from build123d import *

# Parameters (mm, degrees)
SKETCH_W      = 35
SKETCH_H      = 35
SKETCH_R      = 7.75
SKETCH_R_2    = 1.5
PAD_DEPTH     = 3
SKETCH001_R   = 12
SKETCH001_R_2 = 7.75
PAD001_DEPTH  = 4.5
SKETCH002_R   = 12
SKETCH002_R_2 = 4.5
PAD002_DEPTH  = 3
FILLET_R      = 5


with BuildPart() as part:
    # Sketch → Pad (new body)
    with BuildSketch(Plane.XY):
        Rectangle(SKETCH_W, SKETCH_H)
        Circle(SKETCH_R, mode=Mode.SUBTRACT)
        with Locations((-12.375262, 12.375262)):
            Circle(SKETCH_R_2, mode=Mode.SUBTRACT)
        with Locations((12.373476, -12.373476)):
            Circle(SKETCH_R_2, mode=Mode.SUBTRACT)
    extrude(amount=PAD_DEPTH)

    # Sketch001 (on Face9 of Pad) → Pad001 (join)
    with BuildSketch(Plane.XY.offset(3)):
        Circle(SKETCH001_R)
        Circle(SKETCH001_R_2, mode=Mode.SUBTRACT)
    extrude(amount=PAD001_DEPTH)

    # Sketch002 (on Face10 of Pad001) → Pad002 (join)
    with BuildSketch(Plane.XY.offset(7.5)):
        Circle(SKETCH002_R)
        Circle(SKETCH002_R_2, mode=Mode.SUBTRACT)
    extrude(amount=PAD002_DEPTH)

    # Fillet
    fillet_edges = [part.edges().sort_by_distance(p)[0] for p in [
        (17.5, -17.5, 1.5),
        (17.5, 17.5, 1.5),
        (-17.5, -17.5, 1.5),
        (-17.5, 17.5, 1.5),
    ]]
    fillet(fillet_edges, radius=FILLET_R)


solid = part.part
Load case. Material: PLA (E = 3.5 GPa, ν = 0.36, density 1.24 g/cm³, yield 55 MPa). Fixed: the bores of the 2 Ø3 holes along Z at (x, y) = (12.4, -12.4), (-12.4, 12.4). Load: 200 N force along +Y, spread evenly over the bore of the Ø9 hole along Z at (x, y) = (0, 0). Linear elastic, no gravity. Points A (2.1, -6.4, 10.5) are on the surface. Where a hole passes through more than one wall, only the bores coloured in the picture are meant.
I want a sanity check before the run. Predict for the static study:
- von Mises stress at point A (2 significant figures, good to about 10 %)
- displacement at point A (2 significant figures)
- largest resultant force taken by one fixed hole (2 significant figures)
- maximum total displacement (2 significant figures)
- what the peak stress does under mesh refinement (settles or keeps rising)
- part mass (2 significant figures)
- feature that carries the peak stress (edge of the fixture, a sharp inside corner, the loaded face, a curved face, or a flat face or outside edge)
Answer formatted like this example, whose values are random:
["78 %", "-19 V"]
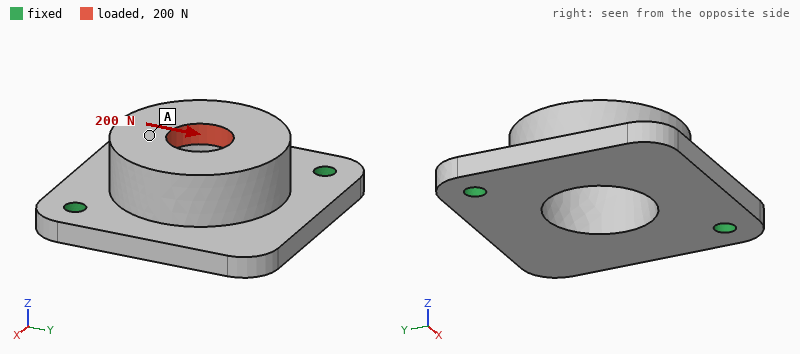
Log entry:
["3.8 MPa", "0.18 mm", "110 N", "0.40 mm", "keeps rising", "6.6 g", "edge of the fixture"]
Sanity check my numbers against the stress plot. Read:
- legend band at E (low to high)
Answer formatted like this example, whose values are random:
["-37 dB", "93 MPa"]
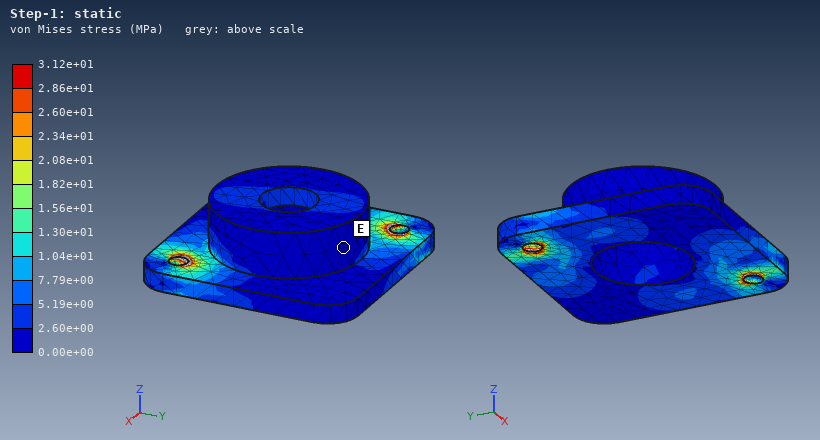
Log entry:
["0.00e+00 to 2.60e+00 MPa"]
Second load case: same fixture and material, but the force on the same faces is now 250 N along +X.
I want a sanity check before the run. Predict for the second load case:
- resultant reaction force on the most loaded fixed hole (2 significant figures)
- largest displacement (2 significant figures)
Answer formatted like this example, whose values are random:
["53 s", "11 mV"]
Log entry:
["130 N", "0.50 mm"]
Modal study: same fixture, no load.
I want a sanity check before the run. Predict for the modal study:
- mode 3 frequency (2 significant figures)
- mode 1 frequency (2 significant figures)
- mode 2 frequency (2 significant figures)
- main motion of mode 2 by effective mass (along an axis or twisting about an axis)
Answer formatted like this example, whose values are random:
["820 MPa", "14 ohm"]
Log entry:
["7000 Hz", "1500 Hz", "3500 Hz", "along Z"]
